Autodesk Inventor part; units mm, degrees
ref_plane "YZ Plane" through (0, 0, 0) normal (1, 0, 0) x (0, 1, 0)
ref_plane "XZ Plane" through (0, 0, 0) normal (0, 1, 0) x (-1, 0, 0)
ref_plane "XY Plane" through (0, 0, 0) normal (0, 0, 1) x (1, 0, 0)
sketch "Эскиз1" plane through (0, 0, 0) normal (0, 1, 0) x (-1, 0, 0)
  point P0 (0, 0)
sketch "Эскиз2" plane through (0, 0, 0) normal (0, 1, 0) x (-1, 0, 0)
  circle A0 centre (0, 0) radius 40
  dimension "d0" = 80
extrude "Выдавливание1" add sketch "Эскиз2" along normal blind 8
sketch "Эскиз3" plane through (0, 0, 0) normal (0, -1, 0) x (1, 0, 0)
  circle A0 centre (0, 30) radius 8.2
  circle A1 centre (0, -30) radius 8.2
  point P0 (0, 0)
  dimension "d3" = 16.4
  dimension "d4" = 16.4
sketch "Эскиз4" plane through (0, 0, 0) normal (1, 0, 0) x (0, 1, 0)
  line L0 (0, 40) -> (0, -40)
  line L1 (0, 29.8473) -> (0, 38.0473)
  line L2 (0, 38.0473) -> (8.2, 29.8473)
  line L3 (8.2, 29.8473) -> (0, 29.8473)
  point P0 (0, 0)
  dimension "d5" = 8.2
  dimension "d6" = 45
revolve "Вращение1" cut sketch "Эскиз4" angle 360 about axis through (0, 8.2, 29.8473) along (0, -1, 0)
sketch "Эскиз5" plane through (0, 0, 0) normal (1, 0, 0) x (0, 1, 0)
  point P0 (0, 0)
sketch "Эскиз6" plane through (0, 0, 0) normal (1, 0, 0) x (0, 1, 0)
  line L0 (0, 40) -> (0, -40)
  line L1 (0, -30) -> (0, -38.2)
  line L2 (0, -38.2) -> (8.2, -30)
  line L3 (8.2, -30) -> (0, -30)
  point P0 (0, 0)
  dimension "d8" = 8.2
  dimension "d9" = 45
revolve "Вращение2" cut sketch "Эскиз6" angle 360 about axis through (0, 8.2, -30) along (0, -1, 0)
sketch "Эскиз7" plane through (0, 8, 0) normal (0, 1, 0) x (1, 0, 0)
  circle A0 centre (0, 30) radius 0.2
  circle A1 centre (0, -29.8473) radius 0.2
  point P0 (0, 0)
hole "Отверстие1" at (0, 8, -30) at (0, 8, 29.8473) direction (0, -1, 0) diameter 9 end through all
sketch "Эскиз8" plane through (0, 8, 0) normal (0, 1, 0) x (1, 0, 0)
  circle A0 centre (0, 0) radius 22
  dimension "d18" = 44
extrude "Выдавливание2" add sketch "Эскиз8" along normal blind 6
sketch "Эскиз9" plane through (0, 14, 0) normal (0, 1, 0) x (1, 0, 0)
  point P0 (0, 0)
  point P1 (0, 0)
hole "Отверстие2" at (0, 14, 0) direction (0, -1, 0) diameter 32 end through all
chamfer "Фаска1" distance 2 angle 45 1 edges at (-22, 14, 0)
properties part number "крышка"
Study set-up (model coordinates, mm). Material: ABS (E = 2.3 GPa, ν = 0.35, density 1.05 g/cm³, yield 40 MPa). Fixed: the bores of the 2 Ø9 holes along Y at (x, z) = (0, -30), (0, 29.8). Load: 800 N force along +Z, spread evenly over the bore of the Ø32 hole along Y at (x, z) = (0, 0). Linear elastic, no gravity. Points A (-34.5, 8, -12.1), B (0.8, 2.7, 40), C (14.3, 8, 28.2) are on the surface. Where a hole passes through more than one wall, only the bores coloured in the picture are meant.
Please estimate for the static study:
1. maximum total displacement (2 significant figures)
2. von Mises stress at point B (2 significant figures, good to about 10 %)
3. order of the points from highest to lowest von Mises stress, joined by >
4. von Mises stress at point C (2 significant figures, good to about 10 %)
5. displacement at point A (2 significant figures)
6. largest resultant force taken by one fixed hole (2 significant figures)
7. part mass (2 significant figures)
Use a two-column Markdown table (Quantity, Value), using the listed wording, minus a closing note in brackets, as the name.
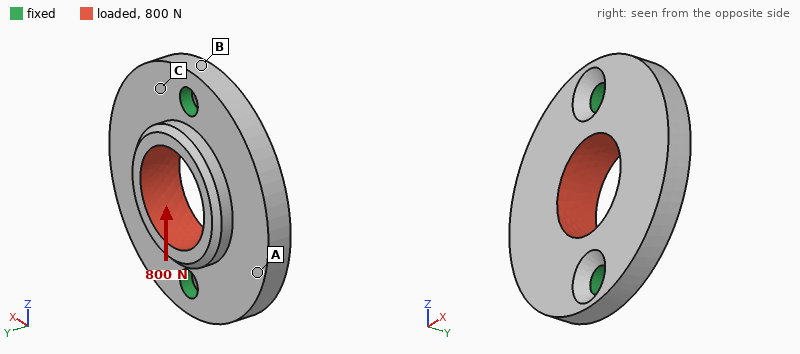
| Quantity | Value |
|---|---|
| maximum total displacement | 33 µm |
| von Mises stress at point B | 1.9 MPa |
| order of the points from highest to lowest von Mises stress, joined by > | B > C > A |
| von Mises stress at point C | 1.1 MPa |
| displacement at point A | 23 µm |
| largest resultant force taken by one fixed hole | 400 N |
| part mass | 38 g |
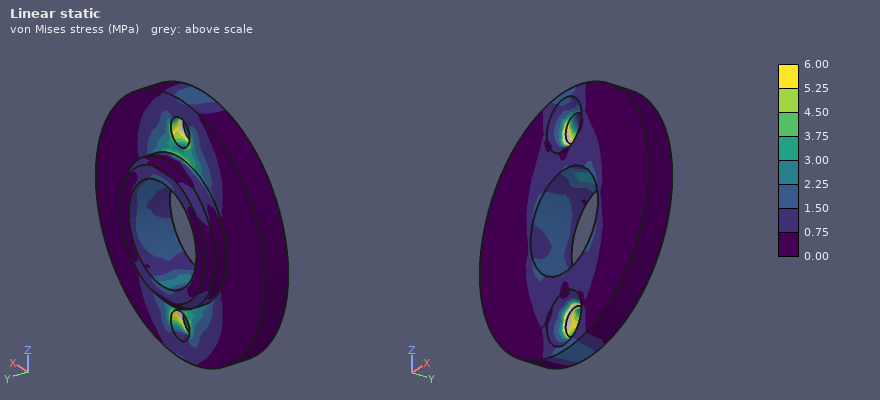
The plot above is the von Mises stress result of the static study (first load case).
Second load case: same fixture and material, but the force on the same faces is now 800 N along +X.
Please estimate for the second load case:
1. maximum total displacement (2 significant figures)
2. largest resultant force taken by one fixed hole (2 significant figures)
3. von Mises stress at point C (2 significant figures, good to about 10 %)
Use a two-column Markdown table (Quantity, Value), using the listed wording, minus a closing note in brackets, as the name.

| Quantity | Value |
|---|---|
| maximum total displacement | 0.10 mm |
| largest resultant force taken by one fixed hole | 400 N |
| von Mises stress at point C | 1.9 MPa |
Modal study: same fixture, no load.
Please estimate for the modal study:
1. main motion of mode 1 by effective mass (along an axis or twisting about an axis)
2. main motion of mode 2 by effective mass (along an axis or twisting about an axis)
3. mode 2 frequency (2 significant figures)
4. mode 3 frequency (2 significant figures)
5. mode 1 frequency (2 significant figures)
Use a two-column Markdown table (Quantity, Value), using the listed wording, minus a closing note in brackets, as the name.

| Quantity | Value |
|---|---|
| main motion of mode 1 by effective mass | twisting about Z |
| main motion of mode 2 by effective mass | along Y |
| mode 2 frequency | 1300 Hz |
| mode 3 frequency | 2700 Hz |
| mode 1 frequency | 930 Hz |
